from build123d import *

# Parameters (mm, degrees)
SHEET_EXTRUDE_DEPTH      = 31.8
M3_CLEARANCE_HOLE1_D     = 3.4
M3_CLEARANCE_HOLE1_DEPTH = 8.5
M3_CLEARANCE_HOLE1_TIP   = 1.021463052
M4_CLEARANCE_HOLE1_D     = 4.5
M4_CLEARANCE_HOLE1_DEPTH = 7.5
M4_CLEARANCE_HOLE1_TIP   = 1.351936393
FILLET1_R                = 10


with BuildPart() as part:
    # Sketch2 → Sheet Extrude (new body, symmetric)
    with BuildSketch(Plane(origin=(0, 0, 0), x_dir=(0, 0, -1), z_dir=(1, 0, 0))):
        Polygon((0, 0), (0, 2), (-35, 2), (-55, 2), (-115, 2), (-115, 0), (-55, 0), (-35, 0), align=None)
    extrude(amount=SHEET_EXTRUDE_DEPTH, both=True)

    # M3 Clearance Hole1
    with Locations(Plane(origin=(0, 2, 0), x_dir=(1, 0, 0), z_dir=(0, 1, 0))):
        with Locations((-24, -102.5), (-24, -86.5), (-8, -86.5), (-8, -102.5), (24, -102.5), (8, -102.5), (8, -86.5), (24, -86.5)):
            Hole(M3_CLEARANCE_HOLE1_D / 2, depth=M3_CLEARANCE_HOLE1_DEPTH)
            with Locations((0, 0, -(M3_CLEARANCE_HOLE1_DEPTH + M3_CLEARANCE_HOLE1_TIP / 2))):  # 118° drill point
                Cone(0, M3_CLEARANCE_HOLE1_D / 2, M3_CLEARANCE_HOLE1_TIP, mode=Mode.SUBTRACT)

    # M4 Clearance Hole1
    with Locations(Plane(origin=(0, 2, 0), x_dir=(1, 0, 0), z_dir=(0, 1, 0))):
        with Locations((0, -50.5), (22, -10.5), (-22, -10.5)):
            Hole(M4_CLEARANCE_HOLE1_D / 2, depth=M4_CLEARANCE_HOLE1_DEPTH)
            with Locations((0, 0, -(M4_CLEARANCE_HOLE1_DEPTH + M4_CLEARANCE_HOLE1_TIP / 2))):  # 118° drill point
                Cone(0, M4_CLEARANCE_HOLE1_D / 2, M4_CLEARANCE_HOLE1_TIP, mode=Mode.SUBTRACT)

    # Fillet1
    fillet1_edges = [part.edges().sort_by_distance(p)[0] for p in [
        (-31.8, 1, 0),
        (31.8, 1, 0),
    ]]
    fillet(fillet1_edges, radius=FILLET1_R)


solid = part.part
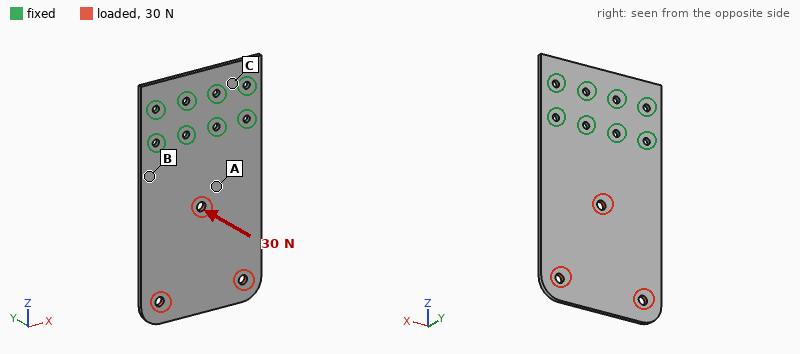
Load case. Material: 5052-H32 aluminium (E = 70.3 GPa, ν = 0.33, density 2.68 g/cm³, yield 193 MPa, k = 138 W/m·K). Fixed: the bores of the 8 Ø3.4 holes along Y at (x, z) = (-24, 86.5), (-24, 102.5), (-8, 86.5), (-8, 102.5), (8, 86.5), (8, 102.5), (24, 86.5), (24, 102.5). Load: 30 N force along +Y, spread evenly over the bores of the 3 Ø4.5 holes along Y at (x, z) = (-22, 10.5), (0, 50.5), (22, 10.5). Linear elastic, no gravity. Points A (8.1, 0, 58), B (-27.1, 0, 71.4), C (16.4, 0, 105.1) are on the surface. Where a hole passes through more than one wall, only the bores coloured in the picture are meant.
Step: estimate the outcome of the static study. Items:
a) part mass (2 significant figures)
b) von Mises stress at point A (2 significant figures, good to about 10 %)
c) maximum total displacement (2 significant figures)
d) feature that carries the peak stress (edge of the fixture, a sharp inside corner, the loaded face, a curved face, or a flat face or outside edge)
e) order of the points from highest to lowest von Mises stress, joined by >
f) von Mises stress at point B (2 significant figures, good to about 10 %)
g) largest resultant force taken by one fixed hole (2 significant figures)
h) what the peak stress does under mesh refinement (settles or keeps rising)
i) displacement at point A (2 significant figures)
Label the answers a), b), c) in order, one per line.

a) 38 g
b) 22 MPa
c) 1.3 mm
d) edge of the fixture
e) B > A > C
f) 33 MPa
g) 21 N
h) keeps rising
i) 0.20 mm
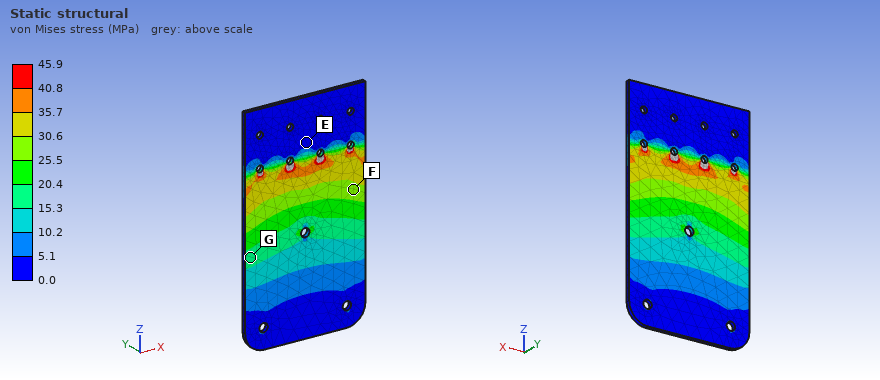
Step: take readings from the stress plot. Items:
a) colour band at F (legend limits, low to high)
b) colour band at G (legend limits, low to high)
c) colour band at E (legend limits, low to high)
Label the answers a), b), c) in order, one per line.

a) 25.5 to 30.6 MPa
b) 15.3 to 20.4 MPa
c) 0.0 to 5.1 MPa
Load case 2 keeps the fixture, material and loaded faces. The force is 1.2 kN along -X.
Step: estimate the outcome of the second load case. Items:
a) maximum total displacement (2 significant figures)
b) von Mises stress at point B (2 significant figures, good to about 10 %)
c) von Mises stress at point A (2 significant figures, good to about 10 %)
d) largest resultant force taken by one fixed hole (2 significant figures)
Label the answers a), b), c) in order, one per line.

a) 89 µm
b) 37 MPa
c) 24 MPa
d) 1.2 kN
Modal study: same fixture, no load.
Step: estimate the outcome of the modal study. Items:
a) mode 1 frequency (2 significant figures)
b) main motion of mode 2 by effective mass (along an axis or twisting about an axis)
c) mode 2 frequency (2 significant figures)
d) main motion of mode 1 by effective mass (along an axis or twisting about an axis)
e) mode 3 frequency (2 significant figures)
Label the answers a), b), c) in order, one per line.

a) 240 Hz
b) twisting about Z
c) 720 Hz
d) along Y
e) 1400 Hz
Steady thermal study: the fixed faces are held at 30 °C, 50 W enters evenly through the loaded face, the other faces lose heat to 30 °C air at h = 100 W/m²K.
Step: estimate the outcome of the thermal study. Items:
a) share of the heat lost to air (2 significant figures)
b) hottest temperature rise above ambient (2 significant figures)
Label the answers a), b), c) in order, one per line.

a) 74 %
b) 75 K
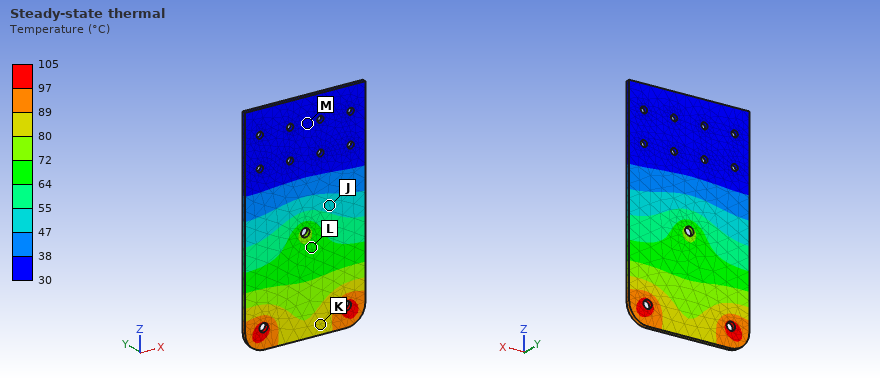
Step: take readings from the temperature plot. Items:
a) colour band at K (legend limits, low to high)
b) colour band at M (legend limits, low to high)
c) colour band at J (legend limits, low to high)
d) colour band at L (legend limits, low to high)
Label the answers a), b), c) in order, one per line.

a) 80 to 89 °C
b) 30 to 38 °C
c) 47 to 55 °C
d) 64 to 72 °C
